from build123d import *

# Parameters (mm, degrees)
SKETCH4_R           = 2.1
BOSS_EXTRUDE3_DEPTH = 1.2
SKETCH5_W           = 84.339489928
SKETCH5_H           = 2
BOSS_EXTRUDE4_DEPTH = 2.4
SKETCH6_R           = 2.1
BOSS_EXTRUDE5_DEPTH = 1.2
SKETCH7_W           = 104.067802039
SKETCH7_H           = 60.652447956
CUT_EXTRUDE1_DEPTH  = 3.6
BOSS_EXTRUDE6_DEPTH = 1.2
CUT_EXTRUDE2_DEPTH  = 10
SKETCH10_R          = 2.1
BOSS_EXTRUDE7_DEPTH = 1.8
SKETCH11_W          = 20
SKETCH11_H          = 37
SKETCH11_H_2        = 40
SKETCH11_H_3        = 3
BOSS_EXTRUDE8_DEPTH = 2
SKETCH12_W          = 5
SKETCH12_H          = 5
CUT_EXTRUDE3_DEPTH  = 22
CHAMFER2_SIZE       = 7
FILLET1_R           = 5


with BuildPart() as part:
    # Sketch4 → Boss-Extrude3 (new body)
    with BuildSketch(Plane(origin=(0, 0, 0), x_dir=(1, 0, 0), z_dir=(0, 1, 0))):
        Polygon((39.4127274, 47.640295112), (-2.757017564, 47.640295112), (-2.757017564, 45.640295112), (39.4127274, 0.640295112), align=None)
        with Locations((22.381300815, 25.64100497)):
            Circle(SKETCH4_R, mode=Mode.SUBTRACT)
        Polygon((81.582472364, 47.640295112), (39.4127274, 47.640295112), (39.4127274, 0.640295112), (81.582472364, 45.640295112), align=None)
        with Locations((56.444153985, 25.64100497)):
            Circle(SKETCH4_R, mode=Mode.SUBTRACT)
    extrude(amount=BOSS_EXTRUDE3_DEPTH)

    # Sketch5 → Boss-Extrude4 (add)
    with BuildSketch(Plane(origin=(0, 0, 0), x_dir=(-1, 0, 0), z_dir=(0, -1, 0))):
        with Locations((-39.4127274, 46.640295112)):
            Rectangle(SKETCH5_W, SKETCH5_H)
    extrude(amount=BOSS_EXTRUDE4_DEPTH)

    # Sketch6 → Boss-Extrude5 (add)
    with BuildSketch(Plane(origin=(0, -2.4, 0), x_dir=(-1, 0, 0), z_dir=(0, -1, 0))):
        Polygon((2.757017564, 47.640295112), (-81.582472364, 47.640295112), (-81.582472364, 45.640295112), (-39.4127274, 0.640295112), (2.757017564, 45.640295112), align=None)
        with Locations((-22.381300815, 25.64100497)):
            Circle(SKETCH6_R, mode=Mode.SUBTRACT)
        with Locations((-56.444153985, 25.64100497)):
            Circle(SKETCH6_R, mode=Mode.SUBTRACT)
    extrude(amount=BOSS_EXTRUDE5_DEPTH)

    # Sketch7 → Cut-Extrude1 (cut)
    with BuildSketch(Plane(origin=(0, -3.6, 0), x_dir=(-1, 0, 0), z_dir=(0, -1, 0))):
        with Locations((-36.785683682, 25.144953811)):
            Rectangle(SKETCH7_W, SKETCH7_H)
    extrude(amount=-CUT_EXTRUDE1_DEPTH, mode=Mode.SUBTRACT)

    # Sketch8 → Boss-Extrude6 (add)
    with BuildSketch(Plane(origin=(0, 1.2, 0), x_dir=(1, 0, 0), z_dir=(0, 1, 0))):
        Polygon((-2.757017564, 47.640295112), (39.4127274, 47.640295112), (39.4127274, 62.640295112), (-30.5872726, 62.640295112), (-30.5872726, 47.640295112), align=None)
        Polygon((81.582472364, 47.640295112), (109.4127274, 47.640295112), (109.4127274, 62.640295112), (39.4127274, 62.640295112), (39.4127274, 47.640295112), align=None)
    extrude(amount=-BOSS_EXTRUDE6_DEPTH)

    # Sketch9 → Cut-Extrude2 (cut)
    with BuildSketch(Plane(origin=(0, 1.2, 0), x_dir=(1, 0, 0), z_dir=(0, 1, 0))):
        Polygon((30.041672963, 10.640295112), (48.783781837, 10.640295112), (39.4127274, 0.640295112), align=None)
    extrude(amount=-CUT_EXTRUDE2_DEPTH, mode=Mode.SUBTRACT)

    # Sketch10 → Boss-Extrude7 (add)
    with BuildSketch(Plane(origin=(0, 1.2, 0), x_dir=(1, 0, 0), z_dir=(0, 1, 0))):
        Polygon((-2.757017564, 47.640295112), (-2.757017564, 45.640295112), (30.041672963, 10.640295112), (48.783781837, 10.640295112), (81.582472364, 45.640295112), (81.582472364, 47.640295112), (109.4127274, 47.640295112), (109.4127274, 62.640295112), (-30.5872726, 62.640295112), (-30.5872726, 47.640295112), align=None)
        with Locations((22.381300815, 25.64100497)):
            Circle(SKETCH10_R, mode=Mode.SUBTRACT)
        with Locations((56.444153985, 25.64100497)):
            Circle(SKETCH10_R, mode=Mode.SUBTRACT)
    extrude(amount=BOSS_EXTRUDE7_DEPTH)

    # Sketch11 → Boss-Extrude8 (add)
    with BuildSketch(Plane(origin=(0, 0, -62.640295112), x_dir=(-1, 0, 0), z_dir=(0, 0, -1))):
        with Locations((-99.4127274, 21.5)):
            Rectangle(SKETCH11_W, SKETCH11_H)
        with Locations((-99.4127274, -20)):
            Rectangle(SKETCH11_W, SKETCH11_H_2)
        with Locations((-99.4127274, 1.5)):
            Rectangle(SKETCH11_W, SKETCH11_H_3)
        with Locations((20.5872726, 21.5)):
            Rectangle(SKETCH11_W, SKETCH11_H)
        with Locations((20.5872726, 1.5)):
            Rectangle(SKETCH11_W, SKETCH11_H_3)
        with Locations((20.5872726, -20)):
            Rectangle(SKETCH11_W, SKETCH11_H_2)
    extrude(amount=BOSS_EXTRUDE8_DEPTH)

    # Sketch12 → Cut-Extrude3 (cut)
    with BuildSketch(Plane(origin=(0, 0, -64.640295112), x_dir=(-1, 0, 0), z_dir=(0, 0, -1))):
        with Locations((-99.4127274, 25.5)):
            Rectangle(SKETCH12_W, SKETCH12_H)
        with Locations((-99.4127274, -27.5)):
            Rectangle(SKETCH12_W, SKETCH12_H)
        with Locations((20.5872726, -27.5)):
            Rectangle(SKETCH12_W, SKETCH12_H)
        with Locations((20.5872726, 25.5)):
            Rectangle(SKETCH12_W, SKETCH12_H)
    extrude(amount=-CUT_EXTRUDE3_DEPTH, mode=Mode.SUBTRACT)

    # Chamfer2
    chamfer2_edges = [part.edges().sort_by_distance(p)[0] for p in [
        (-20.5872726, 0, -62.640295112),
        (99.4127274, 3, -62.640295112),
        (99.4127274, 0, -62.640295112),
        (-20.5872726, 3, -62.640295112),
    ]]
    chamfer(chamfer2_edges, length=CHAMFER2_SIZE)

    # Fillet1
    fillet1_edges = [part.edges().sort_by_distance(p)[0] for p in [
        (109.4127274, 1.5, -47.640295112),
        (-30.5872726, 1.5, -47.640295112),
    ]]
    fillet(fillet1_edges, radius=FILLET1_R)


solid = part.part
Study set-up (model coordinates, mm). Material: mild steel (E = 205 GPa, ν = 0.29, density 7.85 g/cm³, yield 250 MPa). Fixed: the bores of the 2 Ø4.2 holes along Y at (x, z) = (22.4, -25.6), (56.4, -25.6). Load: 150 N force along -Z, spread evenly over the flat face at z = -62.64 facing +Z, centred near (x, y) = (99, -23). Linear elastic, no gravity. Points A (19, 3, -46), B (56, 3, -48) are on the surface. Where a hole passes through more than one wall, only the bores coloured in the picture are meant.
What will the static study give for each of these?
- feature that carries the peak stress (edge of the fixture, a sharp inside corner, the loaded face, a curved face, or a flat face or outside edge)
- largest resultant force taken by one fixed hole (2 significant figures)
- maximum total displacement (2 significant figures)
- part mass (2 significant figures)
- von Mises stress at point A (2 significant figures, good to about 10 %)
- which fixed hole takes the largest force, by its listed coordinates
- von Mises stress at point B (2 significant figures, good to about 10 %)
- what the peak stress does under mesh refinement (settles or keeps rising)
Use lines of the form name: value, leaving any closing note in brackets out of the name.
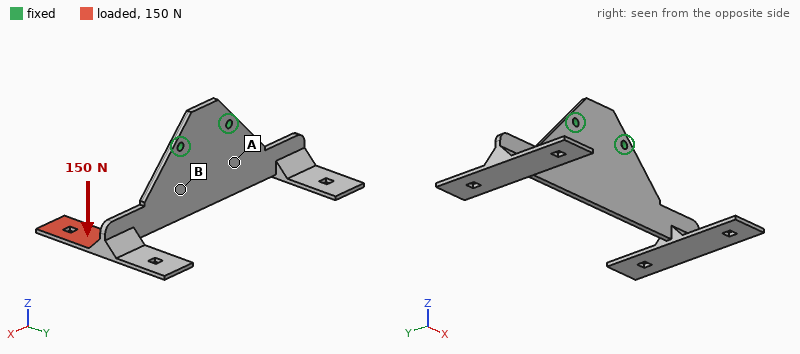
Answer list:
feature that carries the peak stress: a sharp inside corner
largest resultant force taken by one fixed hole: 340 N
maximum total displacement: 0.92 mm
part mass: 160 g
von Mises stress at point A: 18 MPa
which fixed hole takes the largest force, by its listed coordinates: (56.4, -25.6)
von Mises stress at point B: 56 MPa
what the peak stress does under mesh refinement: keeps rising
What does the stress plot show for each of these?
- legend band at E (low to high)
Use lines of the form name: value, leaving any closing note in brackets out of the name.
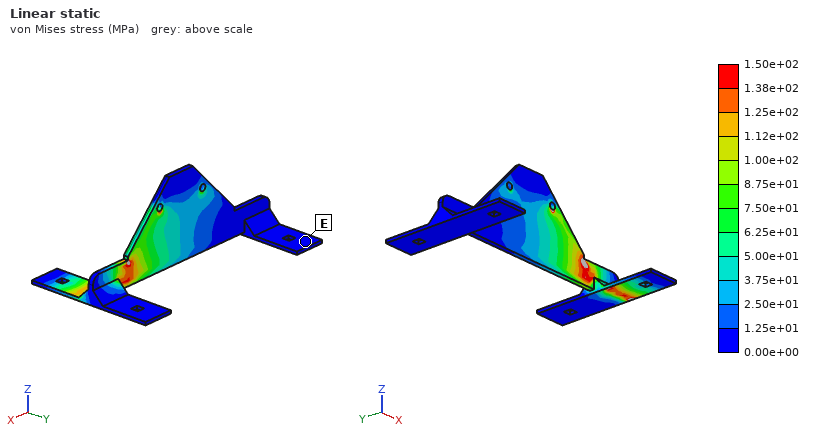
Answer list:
legend band at E: 0.00e+00 to 1.25e+01 MPa
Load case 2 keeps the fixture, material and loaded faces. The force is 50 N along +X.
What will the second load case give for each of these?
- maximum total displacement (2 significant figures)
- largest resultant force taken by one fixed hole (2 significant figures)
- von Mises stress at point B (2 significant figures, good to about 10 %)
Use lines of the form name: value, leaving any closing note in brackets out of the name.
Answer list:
maximum total displacement: 0.30 mm
largest resultant force taken by one fixed hole: 64 N
von Mises stress at point B: 18 MPa
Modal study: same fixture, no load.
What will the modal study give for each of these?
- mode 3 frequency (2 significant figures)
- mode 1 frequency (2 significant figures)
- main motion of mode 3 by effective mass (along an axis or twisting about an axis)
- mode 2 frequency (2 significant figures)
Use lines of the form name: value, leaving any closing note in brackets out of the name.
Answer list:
mode 3 frequency: 640 Hz
mode 1 frequency: 320 Hz
main motion of mode 3 by effective mass: twisting about X
mode 2 frequency: 320 Hz
